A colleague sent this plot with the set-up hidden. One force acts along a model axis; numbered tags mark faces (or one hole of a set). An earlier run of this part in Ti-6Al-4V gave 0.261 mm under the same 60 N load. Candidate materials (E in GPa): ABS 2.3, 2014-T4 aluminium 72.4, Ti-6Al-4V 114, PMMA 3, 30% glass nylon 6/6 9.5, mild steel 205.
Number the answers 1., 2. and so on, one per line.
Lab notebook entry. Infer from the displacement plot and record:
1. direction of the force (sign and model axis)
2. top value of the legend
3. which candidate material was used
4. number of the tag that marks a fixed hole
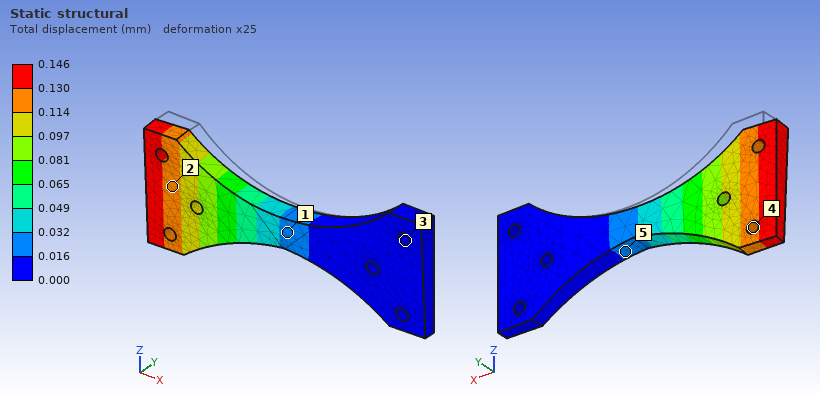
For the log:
1. -Y
2. 0.146 mm
3. mild steel
4. 3
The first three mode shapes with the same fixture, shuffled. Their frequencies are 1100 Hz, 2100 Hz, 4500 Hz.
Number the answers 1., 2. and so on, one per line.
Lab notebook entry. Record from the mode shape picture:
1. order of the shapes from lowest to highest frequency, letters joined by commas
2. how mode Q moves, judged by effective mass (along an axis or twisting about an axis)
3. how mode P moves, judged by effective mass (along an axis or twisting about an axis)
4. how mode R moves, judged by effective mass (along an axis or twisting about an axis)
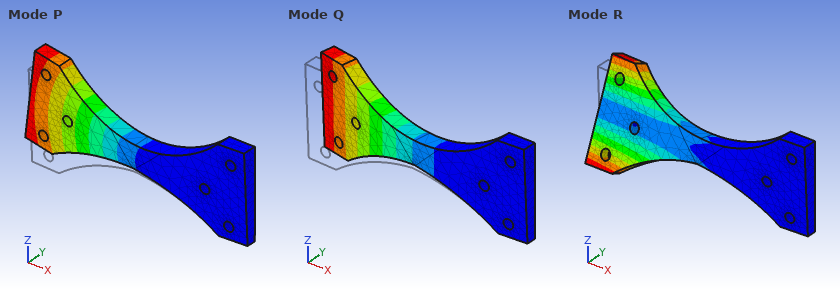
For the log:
1. Q, P, R
2. along Y
3. along Z
4. twisting about X
